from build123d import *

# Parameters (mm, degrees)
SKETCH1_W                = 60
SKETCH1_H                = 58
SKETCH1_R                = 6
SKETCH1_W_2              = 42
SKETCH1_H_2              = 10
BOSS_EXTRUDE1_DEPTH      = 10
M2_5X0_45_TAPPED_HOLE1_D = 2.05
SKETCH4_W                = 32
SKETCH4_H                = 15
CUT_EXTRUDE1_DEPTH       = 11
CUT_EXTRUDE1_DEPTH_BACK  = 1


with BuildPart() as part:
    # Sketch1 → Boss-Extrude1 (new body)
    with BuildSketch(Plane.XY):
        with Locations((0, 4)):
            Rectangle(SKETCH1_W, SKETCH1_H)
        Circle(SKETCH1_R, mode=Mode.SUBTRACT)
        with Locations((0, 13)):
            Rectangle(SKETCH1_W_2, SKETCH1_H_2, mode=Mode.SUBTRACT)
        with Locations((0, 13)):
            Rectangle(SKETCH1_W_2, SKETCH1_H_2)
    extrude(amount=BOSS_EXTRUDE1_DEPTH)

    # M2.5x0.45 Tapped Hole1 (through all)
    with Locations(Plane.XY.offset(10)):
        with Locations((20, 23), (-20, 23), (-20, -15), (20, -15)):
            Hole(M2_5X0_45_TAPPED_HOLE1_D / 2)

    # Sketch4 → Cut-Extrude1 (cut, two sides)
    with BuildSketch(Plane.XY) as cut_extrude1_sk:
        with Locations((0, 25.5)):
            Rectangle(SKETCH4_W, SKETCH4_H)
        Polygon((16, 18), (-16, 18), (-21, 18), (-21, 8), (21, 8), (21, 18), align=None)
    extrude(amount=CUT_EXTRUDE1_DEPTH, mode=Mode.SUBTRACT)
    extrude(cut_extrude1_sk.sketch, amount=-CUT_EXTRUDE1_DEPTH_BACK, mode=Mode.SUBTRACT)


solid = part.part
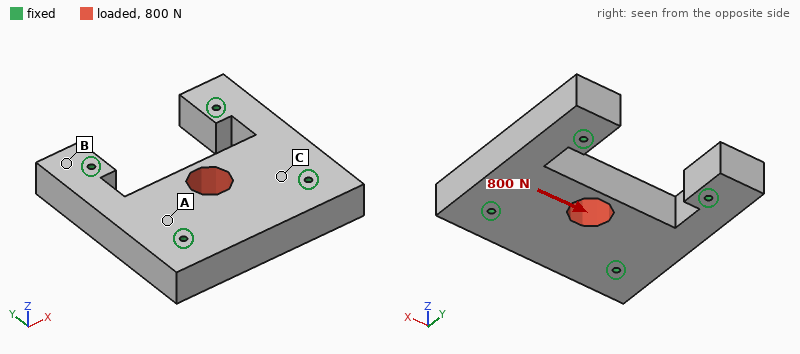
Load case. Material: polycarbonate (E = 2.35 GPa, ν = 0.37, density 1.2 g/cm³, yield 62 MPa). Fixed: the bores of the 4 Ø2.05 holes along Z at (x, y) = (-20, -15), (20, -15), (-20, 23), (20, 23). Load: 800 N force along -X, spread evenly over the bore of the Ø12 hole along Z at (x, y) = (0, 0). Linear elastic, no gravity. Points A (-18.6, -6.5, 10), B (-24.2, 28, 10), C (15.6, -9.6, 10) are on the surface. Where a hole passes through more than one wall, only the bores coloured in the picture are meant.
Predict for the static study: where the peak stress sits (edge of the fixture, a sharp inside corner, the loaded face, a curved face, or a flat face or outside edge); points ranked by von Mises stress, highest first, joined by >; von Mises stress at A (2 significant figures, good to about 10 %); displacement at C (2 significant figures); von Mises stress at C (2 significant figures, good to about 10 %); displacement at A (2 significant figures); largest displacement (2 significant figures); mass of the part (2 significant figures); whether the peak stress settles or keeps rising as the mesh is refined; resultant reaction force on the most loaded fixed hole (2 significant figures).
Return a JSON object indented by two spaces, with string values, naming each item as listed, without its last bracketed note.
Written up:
{
  "where the peak stress sits": "edge of the fixture",
  "points ranked by von Mises stress, highest first, joined by >": "C > A > B",
  "von Mises stress at A": "1.8 MPa",
  "displacement at C": "14 µm",
  "von Mises stress at C": "2.6 MPa",
  "displacement at A": "20 µm",
  "largest displacement": "53 µm",
  "mass of the part": "29 g",
  "whether the peak stress settles or keeps rising as the mesh is refined": "keeps rising",
  "resultant reaction force on the most loaded fixed hole": "360 N"
}
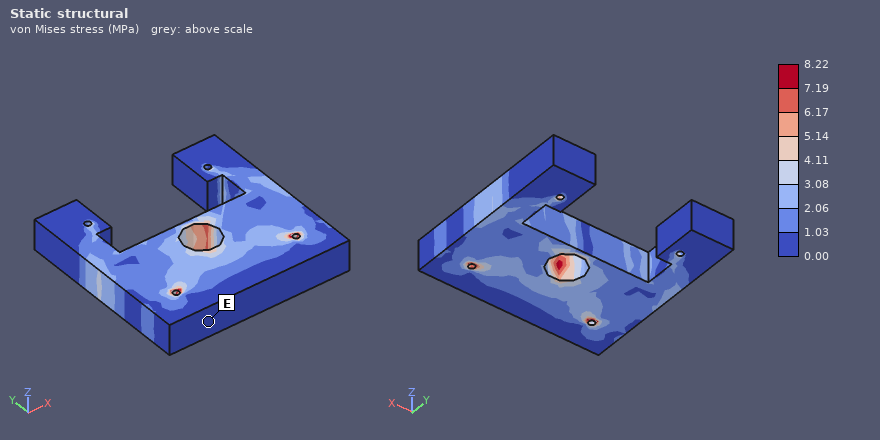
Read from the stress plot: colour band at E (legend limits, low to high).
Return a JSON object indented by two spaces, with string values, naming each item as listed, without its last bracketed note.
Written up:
{
  "colour band at E": "0.00 to 1.03 MPa"
}
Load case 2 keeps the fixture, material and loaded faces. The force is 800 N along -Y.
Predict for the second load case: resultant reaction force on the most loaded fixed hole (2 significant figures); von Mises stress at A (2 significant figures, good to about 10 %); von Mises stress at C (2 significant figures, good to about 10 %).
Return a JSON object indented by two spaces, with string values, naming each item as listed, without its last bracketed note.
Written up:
{
  "resultant reaction force on the most loaded fixed hole": "410 N",
  "von Mises stress at A": "2.3 MPa",
  "von Mises stress at C": "3.6 MPa"
}
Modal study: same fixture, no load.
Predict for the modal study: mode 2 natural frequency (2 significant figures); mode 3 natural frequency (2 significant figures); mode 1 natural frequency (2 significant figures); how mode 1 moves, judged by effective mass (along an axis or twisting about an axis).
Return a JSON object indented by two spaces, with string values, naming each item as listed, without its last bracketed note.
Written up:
{
  "mode 2 natural frequency": "5200 Hz",
  "mode 3 natural frequency": "5400 Hz",
  "mode 1 natural frequency": "3700 Hz",
  "how mode 1 moves, judged by effective mass": "along Z"
}
